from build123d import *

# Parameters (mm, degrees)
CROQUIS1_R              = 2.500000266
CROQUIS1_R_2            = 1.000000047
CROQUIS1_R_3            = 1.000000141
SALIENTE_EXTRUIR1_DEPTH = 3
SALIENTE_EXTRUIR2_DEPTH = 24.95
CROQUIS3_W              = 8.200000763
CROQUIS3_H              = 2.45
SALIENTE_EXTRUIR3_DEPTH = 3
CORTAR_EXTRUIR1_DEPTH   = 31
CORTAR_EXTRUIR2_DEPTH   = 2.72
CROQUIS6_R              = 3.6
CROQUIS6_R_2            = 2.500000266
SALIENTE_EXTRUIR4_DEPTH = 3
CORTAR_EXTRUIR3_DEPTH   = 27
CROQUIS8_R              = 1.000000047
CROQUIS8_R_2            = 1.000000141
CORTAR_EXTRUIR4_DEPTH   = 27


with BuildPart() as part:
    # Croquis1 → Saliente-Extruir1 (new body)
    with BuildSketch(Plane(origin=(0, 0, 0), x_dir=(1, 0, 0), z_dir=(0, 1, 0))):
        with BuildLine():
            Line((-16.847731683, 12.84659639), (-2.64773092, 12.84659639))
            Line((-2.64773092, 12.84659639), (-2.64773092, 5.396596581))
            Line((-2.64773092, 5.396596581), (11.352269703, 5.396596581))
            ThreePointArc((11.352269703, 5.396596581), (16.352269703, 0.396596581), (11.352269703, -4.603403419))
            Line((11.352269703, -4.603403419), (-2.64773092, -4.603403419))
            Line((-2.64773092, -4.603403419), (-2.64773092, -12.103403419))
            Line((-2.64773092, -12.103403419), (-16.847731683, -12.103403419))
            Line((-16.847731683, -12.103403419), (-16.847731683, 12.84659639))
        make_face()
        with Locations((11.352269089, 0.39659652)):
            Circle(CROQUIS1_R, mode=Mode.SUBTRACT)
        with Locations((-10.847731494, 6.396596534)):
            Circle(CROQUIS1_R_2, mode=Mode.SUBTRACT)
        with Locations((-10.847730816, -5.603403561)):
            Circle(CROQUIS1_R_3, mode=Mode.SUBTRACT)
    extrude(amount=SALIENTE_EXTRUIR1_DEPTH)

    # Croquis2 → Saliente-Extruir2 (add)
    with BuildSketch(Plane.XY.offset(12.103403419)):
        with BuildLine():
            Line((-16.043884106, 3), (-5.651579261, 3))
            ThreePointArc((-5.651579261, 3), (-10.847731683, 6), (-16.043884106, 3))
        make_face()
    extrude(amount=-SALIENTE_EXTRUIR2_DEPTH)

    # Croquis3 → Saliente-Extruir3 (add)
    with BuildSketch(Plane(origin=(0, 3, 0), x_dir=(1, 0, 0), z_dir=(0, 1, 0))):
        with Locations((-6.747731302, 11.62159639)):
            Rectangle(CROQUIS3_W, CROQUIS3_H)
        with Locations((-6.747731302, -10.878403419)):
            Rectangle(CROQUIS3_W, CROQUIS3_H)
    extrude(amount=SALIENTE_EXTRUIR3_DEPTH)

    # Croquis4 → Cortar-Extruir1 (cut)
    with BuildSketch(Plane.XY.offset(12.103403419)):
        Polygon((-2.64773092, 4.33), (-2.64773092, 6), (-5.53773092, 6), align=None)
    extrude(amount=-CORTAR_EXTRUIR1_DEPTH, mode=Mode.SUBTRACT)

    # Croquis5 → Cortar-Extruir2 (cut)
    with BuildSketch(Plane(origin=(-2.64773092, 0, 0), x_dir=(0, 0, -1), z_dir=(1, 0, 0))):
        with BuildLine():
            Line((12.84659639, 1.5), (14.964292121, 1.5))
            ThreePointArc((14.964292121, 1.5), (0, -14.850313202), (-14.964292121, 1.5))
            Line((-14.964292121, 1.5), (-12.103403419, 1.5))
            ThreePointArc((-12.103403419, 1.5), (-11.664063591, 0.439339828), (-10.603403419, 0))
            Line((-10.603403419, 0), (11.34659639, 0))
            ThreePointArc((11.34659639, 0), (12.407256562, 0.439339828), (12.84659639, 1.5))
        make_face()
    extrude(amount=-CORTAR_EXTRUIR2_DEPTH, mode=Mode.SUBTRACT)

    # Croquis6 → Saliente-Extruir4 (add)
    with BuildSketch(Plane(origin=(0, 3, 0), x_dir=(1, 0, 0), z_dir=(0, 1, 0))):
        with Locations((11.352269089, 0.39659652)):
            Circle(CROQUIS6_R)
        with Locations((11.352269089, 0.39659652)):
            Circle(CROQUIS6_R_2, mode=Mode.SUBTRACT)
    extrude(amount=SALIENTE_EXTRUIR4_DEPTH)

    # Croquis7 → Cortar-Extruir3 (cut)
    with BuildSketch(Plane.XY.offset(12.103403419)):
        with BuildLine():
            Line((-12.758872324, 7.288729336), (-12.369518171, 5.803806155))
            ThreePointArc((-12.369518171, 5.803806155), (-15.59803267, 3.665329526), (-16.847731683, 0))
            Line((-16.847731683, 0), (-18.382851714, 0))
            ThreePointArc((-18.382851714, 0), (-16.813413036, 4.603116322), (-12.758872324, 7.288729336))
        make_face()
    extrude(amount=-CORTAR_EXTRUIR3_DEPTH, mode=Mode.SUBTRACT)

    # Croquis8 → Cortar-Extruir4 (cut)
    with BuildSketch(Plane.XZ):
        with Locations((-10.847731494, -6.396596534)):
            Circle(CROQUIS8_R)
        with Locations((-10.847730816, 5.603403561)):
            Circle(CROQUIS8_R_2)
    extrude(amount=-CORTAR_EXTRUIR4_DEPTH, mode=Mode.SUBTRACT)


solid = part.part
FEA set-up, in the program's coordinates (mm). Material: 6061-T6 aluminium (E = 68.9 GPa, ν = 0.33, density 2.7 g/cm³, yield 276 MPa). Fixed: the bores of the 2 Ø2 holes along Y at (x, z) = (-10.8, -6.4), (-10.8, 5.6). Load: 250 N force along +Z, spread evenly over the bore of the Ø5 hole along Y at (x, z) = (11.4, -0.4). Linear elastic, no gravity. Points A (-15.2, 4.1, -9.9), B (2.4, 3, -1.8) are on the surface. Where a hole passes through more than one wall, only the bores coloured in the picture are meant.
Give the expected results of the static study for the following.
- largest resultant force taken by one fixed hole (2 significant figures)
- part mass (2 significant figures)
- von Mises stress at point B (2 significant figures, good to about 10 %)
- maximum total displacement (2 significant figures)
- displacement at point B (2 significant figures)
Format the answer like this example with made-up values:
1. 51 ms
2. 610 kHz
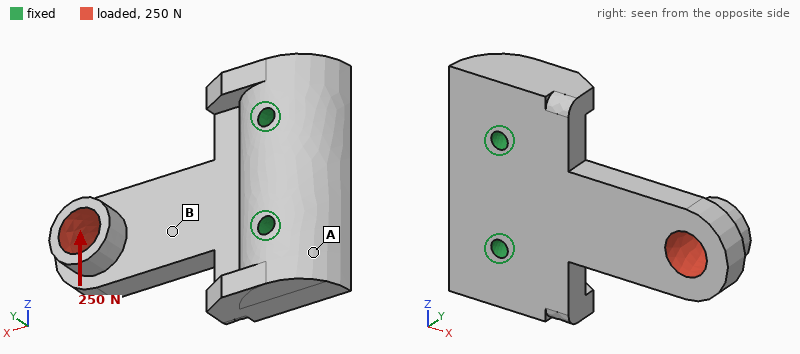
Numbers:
1. 450 N
2. 5.8 g
3. 46 MPa
4. 54 µm
5. 12 µm
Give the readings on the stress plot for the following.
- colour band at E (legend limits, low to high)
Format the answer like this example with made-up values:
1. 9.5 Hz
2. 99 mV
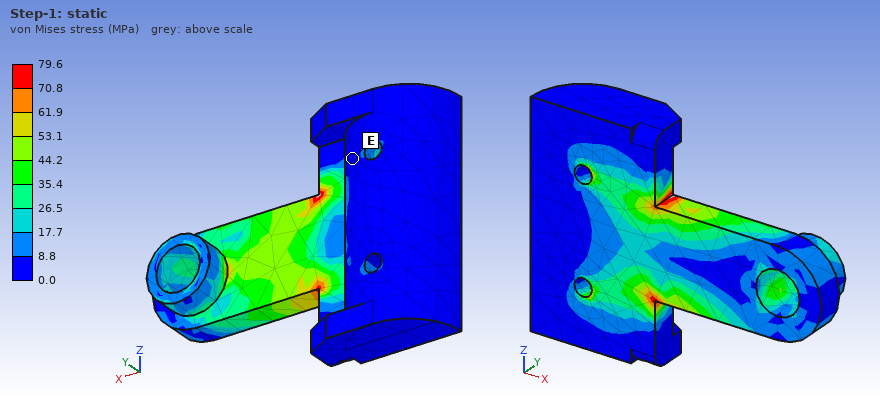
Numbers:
1. 0.0 to 8.8 MPa
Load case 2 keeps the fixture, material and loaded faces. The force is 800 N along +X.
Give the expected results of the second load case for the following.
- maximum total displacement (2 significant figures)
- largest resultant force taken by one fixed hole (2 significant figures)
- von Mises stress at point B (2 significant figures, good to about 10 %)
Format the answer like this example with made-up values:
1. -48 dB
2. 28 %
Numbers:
1. 0.18 mm
2. 420 N
3. 100 MPa
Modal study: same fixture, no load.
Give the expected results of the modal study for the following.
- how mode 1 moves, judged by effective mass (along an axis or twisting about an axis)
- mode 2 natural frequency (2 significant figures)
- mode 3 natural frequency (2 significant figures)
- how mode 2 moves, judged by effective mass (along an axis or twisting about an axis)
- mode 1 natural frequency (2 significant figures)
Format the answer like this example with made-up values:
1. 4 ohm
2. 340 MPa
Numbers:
1. along Y
2. 15 kHz
3. 20 kHz
4. along Z
5. 5000 Hz
